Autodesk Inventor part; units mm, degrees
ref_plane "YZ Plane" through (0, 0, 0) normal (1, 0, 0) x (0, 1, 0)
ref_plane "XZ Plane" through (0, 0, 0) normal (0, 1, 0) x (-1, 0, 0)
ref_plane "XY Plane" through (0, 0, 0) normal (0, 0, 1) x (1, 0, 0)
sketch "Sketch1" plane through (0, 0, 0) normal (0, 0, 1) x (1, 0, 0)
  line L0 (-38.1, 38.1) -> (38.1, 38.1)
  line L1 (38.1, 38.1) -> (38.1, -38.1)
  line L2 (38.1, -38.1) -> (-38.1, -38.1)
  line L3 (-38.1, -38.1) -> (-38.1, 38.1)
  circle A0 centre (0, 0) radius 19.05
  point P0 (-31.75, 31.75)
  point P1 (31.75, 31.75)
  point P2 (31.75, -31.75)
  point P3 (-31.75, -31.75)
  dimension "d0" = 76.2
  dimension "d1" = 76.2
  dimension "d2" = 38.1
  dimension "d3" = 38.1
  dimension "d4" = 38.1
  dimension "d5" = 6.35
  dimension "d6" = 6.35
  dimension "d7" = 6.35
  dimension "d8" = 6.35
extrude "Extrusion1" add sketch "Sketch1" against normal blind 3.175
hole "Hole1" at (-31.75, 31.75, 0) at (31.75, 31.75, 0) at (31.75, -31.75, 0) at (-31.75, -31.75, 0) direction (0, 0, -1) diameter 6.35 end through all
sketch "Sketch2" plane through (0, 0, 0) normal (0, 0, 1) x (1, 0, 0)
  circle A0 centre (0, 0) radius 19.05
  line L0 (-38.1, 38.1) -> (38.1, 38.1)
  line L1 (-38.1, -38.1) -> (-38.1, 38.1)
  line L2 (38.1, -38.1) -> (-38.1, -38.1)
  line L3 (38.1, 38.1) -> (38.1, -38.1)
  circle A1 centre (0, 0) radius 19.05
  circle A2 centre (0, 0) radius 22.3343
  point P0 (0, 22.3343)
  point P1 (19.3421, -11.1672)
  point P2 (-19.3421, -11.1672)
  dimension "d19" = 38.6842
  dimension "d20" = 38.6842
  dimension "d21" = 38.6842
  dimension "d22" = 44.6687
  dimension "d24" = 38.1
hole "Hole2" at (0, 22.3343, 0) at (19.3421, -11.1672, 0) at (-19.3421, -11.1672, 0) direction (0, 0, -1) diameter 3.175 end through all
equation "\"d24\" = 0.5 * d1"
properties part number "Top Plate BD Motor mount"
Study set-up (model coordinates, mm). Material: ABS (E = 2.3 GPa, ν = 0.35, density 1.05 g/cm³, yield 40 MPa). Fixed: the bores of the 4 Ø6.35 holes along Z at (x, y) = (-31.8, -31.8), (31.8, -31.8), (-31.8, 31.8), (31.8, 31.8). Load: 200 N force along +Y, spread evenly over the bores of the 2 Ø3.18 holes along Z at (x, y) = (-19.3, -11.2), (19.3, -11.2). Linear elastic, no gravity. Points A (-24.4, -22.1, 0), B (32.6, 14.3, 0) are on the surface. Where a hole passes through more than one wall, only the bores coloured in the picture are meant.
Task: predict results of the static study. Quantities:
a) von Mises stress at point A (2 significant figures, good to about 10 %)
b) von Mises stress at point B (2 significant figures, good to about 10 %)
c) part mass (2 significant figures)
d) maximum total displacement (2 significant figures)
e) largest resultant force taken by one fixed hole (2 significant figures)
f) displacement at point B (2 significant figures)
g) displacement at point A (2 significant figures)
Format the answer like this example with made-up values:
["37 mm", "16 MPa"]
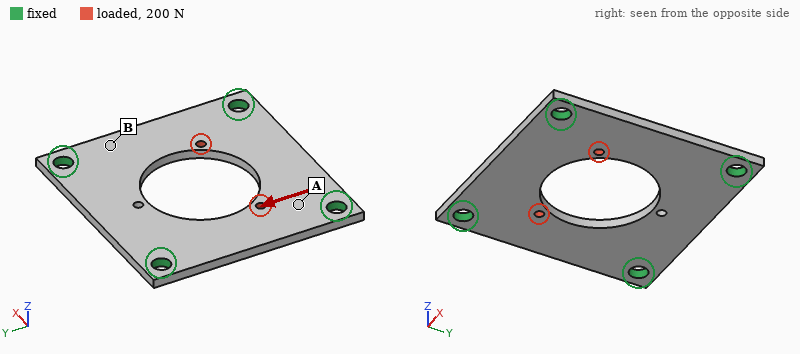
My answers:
["1.5 MPa", "0.68 MPa", "15 g", "26 µm", "70 N", "8.0 µm", "10 µm"]
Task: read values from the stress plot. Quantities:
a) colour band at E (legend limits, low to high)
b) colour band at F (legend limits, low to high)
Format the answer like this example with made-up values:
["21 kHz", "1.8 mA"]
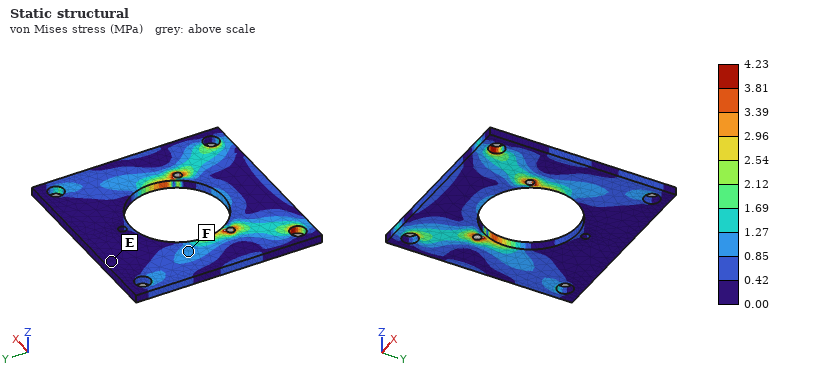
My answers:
["0.00 to 0.42 MPa", "0.85 to 1.27 MPa"]
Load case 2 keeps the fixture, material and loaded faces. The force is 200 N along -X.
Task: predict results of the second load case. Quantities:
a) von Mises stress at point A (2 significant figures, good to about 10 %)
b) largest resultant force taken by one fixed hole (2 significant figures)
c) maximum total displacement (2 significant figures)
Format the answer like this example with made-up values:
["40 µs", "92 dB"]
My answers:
["1.6 MPa", "84 N", "38 µm"]
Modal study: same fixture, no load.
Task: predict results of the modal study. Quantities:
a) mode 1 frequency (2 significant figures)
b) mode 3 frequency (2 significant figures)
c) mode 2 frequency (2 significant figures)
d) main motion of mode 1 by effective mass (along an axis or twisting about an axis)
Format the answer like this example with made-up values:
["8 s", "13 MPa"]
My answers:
["1100 Hz", "1400 Hz", "1400 Hz", "along Z"]
